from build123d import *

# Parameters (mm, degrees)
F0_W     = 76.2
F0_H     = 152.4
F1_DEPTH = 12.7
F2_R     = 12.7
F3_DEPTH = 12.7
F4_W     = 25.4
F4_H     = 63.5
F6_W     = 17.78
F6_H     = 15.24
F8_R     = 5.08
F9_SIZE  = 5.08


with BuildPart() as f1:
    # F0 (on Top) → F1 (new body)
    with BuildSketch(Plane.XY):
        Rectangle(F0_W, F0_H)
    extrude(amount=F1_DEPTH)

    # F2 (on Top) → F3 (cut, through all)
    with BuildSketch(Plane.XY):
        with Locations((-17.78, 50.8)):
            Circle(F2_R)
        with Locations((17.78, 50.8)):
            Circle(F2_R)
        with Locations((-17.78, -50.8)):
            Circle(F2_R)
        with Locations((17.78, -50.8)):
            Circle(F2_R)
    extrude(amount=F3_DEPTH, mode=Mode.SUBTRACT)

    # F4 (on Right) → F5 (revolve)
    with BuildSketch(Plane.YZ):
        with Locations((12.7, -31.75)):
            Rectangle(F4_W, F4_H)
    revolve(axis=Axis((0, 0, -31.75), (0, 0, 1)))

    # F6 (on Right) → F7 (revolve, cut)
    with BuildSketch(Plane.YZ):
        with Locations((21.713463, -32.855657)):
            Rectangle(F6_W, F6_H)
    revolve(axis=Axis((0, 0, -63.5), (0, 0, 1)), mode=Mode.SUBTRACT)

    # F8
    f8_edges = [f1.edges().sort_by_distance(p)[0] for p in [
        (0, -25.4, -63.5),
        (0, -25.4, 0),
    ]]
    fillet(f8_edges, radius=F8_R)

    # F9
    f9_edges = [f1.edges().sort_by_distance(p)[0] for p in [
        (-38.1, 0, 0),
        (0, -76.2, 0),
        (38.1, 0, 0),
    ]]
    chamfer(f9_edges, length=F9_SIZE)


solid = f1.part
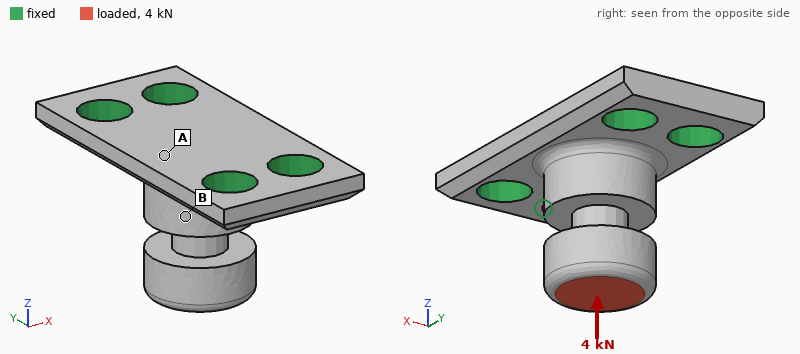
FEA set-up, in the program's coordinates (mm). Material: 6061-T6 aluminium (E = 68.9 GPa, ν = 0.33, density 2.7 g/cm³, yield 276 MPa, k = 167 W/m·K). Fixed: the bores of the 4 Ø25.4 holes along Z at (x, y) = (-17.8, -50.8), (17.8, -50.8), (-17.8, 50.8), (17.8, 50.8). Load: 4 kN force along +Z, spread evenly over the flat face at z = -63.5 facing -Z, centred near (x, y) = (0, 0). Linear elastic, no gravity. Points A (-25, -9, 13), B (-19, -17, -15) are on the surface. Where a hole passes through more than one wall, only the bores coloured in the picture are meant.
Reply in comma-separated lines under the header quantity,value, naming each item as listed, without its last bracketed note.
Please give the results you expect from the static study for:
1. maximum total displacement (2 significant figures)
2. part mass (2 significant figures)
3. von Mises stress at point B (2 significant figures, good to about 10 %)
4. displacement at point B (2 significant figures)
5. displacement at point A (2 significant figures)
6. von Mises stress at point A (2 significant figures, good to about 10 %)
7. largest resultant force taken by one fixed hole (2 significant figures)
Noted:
quantity,value
maximum total displacement,9.5 µm
part mass,600 g
von Mises stress at point B,1.2 MPa
displacement at point B,5.4 µm
displacement at point A,5.3 µm
von Mises stress at point A,4.0 MPa
largest resultant force taken by one fixed hole,1.1 kN
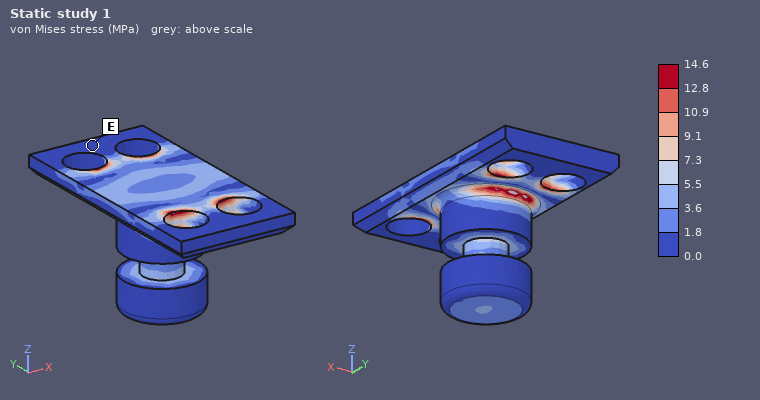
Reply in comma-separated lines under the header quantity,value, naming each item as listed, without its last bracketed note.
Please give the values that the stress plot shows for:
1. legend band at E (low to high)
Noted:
quantity,value
legend band at E,0.0 to 1.8 MPa
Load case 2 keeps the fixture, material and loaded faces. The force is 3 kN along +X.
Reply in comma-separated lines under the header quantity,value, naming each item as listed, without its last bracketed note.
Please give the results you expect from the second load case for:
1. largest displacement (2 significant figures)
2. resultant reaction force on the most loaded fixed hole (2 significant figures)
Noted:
quantity,value
largest displacement,0.13 mm
resultant reaction force on the most loaded fixed hole,2.6 kN
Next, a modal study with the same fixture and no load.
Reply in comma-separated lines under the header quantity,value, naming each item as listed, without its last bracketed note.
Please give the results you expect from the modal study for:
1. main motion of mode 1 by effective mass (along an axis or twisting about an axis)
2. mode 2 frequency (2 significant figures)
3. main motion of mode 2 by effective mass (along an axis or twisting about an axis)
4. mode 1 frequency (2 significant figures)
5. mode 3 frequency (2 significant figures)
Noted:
quantity,value
main motion of mode 1 by effective mass,along X
mode 2 frequency,3400 Hz
main motion of mode 2 by effective mass,along Y
mode 1 frequency,2700 Hz
mode 3 frequency,5400 Hz
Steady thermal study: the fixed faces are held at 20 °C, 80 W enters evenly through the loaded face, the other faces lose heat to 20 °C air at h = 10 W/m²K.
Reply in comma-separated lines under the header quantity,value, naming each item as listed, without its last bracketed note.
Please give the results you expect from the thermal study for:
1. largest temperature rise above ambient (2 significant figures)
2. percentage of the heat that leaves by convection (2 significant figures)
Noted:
quantity,value
largest temperature rise above ambient,39 K
percentage of the heat that leaves by convection,4.0 %
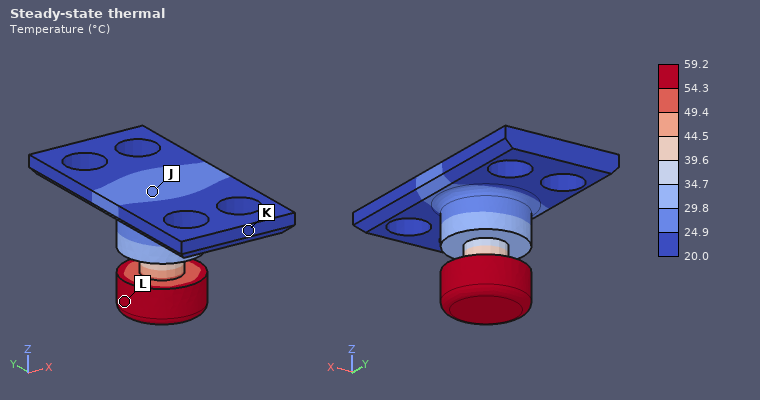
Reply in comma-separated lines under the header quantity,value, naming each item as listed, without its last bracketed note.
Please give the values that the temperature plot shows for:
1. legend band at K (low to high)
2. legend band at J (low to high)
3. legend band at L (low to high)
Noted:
quantity,value
legend band at K,20.0 to 24.9 °C
legend band at J,24.9 to 29.8 °C
legend band at L,54.3 to 59.2 °C
